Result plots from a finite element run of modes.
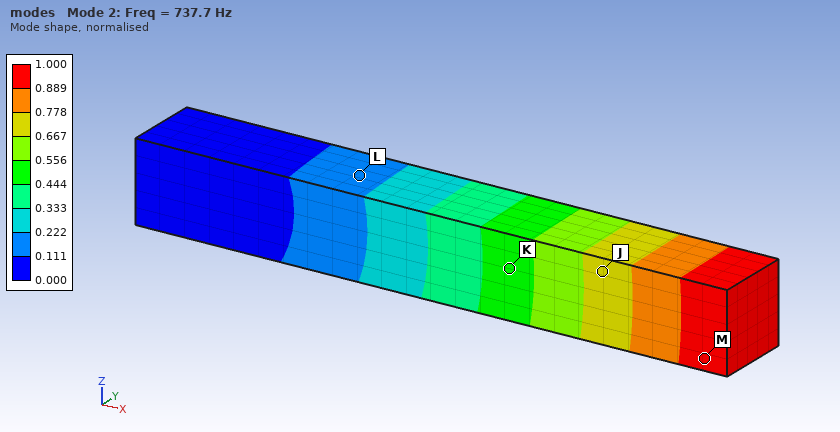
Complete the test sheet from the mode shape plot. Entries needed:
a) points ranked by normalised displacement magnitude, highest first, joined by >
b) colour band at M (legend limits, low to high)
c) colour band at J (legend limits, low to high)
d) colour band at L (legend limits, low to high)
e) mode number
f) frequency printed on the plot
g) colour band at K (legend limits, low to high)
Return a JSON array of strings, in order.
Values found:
["M > J > K > L", "0.889 to 1.000", "0.667 to 0.778", "0.111 to 0.222", "2", "737.7 Hz", "0.444 to 0.556"]
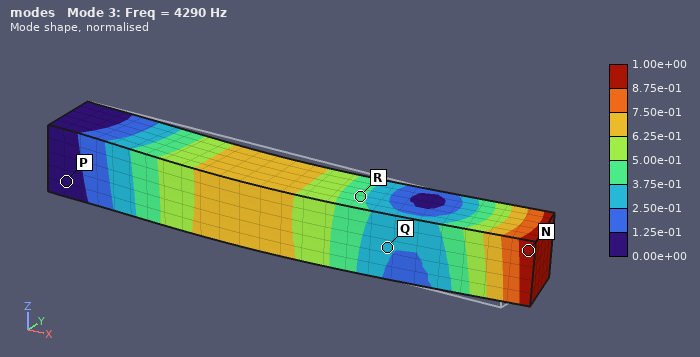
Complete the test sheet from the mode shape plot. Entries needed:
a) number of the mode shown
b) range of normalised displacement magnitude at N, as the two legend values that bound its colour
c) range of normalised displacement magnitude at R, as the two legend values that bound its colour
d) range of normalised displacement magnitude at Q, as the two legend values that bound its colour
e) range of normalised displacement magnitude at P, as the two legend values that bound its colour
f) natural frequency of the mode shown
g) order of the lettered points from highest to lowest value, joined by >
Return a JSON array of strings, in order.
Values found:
["3", "8.75e-01 to 1.00e+00", "3.75e-01 to 5.00e-01", "2.50e-01 to 3.75e-01", "0.00e+00 to 1.25e-01", "4290 Hz", "N > R > Q > P"]
